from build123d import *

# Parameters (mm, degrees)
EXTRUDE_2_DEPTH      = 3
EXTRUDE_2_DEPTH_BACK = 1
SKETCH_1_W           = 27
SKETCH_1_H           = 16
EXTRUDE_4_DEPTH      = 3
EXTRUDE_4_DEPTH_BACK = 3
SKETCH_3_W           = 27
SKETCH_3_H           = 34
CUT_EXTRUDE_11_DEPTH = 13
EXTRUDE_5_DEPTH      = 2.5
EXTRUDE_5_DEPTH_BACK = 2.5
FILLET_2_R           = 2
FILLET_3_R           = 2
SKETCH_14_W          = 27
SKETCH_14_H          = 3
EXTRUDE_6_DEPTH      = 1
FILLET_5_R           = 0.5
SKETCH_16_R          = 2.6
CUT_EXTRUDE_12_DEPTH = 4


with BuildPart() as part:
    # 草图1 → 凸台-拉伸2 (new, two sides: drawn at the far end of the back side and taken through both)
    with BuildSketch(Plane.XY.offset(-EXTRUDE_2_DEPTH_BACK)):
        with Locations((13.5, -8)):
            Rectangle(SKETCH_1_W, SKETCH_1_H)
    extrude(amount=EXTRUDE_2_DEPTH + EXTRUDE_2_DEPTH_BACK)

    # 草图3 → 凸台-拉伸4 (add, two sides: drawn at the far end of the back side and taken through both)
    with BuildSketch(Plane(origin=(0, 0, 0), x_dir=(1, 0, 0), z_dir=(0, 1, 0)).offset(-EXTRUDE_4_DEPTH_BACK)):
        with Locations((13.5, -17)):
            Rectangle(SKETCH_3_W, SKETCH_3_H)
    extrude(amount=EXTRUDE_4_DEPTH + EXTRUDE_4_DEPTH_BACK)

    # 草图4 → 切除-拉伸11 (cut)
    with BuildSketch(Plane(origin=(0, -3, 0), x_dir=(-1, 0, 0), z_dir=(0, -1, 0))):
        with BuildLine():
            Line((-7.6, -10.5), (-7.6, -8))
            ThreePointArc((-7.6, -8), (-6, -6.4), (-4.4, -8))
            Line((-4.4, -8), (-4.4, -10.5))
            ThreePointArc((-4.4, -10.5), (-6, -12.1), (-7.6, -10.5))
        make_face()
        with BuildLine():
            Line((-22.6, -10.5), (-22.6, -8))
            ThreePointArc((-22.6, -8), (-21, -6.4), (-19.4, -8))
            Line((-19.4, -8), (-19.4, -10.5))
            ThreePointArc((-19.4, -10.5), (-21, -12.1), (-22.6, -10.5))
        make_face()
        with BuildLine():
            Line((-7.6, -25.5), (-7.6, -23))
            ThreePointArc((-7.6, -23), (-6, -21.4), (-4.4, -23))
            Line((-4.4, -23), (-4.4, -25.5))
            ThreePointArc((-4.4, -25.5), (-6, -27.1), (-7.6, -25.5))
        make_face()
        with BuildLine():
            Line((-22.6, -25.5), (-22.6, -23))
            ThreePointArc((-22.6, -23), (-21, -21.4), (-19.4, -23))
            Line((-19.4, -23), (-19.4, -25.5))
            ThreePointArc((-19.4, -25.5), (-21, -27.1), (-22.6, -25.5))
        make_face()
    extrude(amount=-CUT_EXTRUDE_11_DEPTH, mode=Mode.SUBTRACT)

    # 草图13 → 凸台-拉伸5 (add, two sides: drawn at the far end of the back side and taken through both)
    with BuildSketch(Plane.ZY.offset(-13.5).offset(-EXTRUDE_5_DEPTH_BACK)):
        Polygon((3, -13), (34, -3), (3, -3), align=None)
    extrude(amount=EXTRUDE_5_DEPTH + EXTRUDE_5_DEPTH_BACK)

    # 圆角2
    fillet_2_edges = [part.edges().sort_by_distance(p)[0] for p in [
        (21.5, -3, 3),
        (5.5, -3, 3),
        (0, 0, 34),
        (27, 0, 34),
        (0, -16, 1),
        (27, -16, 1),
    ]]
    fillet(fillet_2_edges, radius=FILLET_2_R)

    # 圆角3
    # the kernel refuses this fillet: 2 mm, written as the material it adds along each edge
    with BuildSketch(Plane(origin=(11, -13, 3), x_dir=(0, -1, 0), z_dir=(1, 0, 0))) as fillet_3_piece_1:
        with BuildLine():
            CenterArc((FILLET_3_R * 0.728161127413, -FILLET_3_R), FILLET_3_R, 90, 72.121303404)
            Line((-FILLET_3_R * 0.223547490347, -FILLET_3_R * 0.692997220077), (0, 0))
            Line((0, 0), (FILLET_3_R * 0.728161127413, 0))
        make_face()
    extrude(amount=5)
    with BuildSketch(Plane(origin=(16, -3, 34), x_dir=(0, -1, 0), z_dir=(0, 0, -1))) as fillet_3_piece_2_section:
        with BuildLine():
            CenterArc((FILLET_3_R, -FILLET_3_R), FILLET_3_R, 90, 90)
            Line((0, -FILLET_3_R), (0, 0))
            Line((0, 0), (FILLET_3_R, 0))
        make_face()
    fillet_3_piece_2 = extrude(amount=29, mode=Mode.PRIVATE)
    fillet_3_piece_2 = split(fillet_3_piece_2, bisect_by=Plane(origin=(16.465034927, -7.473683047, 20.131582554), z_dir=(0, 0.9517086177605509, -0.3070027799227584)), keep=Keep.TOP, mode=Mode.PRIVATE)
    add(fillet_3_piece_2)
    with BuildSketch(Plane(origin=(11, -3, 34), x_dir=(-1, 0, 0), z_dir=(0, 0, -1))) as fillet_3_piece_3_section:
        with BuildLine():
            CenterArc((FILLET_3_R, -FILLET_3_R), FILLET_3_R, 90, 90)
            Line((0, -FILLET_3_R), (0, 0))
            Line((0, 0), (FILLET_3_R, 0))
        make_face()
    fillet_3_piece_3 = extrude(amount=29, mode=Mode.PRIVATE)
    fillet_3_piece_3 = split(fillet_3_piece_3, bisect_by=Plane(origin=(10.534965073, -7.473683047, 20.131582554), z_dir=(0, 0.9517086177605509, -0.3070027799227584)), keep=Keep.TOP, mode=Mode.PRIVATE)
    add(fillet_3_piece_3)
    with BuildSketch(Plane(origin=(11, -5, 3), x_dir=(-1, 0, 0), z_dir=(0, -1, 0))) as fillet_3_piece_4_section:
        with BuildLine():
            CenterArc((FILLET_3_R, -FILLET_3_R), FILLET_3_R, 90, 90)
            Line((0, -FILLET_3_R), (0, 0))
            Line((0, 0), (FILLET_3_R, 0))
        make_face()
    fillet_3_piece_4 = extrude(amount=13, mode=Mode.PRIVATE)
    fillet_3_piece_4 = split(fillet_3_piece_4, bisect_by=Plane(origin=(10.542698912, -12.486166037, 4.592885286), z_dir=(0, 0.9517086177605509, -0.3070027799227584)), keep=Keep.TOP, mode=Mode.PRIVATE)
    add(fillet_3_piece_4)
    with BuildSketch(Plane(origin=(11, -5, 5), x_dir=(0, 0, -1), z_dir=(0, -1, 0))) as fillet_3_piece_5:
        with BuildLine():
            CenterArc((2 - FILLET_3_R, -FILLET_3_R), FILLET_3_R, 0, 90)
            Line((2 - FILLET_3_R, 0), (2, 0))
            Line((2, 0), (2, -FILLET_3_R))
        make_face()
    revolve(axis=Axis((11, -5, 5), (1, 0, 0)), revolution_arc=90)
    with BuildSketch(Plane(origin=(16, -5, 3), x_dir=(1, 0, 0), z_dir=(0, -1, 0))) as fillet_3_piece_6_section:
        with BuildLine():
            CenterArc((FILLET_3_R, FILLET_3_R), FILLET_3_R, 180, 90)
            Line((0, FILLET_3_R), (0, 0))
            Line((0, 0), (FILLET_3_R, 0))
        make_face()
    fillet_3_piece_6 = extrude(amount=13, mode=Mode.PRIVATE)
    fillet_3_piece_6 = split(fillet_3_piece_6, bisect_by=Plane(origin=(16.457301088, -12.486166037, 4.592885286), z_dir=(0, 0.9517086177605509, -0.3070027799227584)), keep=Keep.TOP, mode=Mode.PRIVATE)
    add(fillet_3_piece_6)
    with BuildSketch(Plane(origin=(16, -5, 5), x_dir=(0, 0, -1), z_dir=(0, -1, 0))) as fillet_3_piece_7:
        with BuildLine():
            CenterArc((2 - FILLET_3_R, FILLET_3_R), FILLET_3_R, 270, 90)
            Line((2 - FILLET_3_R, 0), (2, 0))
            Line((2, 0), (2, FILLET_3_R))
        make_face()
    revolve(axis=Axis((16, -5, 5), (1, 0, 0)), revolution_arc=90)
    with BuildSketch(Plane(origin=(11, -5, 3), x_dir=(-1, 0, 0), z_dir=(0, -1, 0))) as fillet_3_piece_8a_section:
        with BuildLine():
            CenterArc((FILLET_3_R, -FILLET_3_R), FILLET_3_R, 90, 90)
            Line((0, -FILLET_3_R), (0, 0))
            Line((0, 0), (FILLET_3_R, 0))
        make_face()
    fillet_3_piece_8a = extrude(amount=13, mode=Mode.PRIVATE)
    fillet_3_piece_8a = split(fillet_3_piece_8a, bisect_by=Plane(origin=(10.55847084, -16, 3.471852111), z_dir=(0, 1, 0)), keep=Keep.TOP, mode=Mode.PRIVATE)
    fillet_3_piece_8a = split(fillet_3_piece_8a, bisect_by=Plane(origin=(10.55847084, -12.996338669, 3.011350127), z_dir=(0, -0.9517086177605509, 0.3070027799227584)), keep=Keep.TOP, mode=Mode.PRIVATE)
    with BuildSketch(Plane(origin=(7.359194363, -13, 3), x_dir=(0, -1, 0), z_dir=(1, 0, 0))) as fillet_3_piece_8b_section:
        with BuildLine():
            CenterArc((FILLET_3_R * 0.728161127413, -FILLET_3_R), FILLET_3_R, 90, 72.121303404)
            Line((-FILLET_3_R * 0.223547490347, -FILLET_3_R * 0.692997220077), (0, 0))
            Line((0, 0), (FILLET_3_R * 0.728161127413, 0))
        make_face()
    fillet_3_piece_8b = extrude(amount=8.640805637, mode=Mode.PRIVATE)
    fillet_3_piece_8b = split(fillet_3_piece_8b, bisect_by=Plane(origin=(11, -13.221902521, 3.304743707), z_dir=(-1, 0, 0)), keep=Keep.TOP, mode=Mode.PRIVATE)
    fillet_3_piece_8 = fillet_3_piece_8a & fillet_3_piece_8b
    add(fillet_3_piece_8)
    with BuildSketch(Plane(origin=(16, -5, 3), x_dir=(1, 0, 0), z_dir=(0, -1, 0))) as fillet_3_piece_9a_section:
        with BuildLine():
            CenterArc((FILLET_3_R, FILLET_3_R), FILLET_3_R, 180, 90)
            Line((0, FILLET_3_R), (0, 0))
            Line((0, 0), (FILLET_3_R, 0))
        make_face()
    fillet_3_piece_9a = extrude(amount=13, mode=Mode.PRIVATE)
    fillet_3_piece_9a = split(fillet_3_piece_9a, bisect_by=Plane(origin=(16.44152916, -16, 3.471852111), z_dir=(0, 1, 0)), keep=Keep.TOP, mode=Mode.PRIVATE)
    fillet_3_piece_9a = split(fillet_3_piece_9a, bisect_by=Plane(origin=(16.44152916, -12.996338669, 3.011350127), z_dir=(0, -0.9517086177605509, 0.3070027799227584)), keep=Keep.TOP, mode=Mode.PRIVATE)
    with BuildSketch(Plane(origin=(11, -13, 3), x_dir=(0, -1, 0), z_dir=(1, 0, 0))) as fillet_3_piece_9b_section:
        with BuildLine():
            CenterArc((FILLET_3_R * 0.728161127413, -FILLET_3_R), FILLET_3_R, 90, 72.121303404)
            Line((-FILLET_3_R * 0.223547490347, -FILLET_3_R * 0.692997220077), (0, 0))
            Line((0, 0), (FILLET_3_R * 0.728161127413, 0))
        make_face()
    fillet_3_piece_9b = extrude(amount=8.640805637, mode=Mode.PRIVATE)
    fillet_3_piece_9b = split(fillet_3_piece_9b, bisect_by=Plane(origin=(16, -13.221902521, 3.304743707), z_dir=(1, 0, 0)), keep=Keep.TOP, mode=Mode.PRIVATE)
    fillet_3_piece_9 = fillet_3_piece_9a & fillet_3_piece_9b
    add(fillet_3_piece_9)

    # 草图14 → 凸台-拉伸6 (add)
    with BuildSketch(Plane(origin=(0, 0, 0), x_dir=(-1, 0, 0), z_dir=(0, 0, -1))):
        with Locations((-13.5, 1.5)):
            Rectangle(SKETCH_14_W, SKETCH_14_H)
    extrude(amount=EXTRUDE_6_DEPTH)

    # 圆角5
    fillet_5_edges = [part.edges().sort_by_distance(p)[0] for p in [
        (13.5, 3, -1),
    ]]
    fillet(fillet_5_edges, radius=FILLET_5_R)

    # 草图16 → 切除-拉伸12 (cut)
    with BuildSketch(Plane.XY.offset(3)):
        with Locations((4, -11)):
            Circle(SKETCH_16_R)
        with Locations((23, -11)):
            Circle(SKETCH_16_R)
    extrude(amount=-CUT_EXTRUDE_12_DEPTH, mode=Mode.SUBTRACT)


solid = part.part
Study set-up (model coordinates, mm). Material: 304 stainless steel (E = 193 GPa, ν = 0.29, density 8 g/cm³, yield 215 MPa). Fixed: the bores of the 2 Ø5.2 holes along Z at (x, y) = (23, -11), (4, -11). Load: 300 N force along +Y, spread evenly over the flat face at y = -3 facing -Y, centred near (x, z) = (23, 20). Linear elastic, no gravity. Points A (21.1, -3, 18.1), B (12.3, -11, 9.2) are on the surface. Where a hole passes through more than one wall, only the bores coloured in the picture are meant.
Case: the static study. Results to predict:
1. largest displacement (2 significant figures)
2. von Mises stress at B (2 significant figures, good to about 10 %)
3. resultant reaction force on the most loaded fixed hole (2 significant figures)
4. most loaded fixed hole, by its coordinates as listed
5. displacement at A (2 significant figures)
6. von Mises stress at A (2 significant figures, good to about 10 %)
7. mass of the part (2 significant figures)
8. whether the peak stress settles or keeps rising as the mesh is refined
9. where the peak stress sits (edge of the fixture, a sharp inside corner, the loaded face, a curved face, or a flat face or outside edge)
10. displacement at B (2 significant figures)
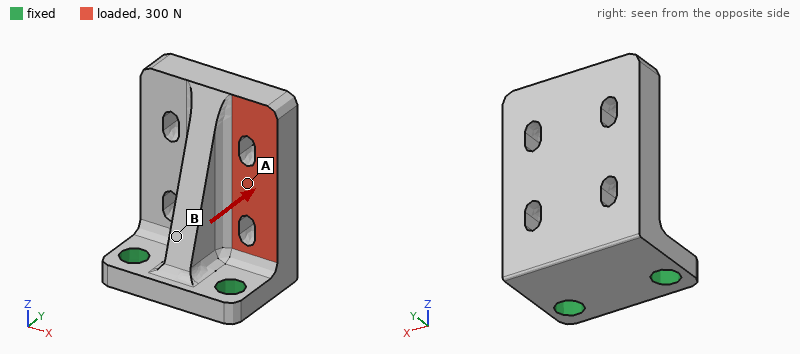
29 µm
24 MPa
290 N
(23, -11)
14 µm
11 MPa
59 g
keeps rising
a sharp inside corner
5.5 µm
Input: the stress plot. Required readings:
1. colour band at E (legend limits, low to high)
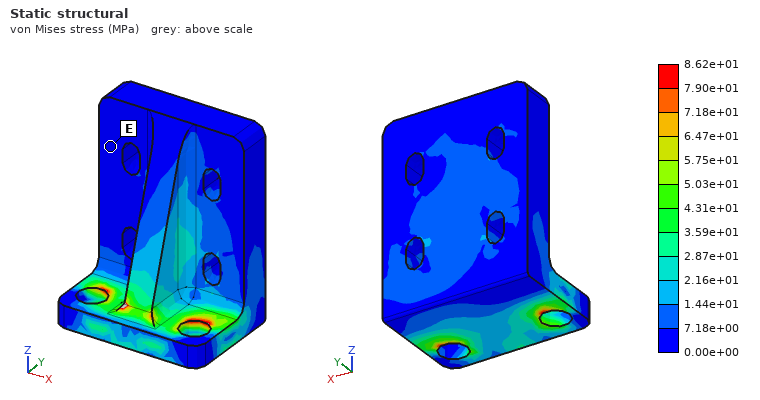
0.00e+00 to 7.18e+00 MPa
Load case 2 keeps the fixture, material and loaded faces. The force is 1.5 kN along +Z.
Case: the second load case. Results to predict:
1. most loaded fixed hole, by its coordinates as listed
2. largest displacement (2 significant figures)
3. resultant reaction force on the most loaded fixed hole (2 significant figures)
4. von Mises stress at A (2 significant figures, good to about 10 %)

(23, -11)
36 µm
1.5 kN
23 MPa
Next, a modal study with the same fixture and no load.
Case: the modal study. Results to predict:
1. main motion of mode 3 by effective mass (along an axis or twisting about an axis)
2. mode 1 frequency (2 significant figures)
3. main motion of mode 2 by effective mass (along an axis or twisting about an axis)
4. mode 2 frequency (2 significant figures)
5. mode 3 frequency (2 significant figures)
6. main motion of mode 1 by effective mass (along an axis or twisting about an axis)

twisting about Z
3300 Hz
along X
5900 Hz
11 kHz
along Y
